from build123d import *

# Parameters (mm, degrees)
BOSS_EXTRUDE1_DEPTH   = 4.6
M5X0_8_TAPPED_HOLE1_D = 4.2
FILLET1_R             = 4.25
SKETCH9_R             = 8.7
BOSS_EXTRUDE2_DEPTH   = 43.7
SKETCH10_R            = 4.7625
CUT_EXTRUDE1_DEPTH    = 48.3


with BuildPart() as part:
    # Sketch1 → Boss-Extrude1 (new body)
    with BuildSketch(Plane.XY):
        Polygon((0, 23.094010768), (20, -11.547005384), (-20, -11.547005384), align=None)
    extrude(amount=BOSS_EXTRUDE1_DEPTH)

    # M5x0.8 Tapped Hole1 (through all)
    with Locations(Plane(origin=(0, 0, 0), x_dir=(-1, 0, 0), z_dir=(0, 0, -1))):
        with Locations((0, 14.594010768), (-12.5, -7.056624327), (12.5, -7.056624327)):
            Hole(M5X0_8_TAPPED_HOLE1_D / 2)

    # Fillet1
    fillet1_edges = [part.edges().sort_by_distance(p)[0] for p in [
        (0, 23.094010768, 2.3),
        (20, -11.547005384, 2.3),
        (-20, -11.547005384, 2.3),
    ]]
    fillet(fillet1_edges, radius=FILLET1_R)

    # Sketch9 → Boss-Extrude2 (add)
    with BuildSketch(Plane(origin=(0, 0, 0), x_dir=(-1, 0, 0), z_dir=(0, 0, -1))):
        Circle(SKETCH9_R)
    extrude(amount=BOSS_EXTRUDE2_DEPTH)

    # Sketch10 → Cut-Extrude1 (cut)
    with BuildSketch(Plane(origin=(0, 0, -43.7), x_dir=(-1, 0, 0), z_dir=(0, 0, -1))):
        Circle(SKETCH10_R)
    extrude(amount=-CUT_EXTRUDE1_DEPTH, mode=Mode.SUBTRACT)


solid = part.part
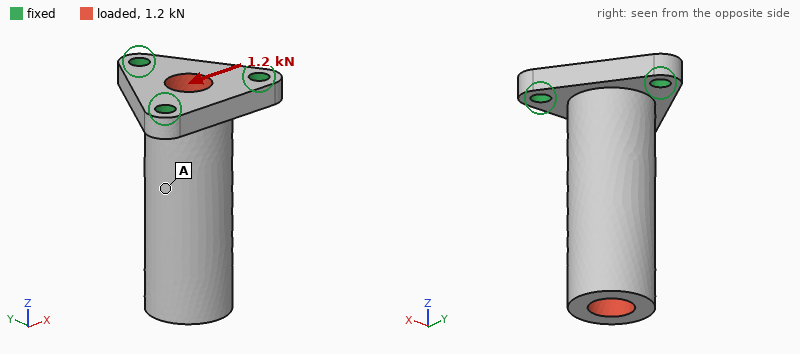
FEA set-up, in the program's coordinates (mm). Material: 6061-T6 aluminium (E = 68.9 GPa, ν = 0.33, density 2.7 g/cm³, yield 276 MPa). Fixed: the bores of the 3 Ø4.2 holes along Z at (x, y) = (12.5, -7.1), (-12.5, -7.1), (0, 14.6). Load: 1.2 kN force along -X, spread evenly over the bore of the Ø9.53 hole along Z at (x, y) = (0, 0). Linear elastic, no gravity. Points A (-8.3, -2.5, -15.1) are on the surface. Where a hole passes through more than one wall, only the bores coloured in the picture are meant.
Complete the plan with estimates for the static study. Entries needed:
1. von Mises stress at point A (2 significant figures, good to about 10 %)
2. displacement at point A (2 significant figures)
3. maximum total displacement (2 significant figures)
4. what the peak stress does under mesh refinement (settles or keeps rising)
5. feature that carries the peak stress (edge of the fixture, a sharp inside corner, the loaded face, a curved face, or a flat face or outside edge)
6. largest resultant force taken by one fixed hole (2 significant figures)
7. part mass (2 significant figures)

20 MPa
0.042 mm
0.12 mm
keeps rising
edge of the fixture
1.3 kN
26 g
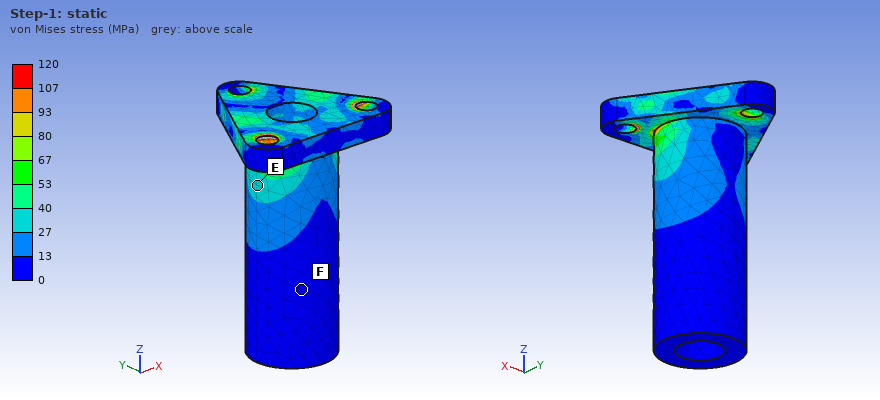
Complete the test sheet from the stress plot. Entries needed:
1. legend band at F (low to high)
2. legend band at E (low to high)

0 to 13 MPa
27 to 40 MPa
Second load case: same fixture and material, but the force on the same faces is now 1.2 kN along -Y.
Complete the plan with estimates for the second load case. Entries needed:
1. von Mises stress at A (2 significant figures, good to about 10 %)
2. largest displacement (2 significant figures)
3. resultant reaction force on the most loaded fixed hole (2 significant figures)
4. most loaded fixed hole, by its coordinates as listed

13 MPa
0.12 mm
1.5 kN
(0, 14.6)
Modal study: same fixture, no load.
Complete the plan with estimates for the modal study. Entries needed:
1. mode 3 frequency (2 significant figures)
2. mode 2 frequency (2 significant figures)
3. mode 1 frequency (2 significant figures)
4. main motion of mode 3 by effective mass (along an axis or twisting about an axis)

16 kHz
4200 Hz
4200 Hz
along Z
